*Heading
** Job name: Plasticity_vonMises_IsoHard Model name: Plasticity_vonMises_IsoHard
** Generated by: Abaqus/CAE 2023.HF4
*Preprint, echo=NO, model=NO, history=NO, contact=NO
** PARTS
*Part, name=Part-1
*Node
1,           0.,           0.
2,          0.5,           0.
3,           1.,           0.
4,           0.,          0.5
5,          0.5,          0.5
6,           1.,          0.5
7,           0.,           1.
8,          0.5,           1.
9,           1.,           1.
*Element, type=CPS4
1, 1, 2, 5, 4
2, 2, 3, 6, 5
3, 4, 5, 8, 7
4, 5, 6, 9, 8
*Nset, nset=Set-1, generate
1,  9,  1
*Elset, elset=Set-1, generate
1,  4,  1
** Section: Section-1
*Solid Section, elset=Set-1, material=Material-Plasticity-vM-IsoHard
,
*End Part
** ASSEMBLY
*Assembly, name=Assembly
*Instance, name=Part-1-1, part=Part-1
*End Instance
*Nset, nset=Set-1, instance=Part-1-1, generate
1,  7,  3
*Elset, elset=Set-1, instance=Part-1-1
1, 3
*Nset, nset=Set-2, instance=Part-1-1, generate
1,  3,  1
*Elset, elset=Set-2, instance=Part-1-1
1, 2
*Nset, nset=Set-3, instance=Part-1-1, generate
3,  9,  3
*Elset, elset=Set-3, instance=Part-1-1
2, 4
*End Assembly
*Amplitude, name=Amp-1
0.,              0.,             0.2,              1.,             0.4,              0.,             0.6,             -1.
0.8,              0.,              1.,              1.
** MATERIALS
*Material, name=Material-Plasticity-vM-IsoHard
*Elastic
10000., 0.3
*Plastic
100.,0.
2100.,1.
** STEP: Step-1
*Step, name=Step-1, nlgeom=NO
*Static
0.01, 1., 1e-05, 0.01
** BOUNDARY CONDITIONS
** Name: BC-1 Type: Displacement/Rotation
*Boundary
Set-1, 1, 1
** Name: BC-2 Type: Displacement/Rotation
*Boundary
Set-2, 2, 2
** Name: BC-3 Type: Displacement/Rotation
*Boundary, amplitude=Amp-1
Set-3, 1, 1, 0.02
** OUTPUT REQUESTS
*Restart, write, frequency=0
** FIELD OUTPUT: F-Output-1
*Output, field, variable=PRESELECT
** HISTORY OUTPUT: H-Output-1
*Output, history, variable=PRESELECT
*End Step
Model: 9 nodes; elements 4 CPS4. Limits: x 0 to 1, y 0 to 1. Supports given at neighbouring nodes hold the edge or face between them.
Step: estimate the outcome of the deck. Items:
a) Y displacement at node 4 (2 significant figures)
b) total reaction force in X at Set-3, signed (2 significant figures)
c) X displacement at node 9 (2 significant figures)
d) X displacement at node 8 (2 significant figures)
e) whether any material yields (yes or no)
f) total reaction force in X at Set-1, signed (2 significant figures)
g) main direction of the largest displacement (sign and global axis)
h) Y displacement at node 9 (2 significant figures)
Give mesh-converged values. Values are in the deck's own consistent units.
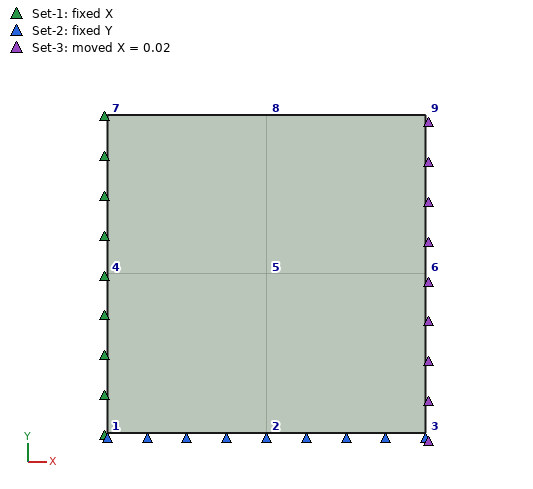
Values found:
-0.0034
160
0.020
0.010
yes
-160
+X
-0.0068
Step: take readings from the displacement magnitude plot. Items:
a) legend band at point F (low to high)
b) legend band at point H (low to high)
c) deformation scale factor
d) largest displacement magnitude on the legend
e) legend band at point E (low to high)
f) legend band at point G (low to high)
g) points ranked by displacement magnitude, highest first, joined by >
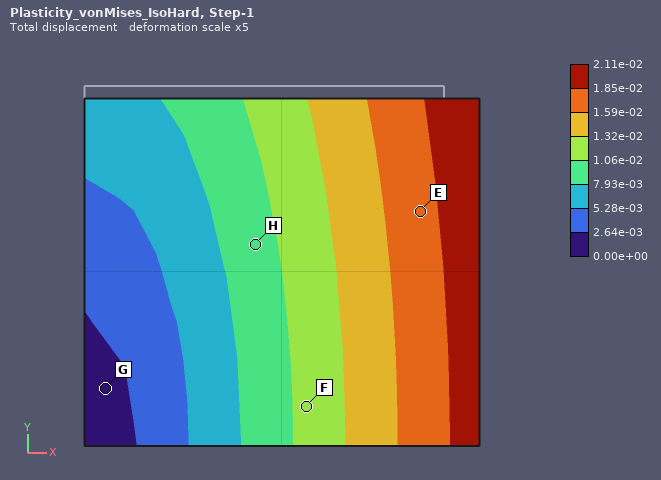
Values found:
1.06e-02 to 1.32e-02
7.93e-03 to 1.06e-02
5
2.11e-02
1.59e-02 to 1.85e-02
0.00e+00 to 2.64e-03
E > F > H > G
